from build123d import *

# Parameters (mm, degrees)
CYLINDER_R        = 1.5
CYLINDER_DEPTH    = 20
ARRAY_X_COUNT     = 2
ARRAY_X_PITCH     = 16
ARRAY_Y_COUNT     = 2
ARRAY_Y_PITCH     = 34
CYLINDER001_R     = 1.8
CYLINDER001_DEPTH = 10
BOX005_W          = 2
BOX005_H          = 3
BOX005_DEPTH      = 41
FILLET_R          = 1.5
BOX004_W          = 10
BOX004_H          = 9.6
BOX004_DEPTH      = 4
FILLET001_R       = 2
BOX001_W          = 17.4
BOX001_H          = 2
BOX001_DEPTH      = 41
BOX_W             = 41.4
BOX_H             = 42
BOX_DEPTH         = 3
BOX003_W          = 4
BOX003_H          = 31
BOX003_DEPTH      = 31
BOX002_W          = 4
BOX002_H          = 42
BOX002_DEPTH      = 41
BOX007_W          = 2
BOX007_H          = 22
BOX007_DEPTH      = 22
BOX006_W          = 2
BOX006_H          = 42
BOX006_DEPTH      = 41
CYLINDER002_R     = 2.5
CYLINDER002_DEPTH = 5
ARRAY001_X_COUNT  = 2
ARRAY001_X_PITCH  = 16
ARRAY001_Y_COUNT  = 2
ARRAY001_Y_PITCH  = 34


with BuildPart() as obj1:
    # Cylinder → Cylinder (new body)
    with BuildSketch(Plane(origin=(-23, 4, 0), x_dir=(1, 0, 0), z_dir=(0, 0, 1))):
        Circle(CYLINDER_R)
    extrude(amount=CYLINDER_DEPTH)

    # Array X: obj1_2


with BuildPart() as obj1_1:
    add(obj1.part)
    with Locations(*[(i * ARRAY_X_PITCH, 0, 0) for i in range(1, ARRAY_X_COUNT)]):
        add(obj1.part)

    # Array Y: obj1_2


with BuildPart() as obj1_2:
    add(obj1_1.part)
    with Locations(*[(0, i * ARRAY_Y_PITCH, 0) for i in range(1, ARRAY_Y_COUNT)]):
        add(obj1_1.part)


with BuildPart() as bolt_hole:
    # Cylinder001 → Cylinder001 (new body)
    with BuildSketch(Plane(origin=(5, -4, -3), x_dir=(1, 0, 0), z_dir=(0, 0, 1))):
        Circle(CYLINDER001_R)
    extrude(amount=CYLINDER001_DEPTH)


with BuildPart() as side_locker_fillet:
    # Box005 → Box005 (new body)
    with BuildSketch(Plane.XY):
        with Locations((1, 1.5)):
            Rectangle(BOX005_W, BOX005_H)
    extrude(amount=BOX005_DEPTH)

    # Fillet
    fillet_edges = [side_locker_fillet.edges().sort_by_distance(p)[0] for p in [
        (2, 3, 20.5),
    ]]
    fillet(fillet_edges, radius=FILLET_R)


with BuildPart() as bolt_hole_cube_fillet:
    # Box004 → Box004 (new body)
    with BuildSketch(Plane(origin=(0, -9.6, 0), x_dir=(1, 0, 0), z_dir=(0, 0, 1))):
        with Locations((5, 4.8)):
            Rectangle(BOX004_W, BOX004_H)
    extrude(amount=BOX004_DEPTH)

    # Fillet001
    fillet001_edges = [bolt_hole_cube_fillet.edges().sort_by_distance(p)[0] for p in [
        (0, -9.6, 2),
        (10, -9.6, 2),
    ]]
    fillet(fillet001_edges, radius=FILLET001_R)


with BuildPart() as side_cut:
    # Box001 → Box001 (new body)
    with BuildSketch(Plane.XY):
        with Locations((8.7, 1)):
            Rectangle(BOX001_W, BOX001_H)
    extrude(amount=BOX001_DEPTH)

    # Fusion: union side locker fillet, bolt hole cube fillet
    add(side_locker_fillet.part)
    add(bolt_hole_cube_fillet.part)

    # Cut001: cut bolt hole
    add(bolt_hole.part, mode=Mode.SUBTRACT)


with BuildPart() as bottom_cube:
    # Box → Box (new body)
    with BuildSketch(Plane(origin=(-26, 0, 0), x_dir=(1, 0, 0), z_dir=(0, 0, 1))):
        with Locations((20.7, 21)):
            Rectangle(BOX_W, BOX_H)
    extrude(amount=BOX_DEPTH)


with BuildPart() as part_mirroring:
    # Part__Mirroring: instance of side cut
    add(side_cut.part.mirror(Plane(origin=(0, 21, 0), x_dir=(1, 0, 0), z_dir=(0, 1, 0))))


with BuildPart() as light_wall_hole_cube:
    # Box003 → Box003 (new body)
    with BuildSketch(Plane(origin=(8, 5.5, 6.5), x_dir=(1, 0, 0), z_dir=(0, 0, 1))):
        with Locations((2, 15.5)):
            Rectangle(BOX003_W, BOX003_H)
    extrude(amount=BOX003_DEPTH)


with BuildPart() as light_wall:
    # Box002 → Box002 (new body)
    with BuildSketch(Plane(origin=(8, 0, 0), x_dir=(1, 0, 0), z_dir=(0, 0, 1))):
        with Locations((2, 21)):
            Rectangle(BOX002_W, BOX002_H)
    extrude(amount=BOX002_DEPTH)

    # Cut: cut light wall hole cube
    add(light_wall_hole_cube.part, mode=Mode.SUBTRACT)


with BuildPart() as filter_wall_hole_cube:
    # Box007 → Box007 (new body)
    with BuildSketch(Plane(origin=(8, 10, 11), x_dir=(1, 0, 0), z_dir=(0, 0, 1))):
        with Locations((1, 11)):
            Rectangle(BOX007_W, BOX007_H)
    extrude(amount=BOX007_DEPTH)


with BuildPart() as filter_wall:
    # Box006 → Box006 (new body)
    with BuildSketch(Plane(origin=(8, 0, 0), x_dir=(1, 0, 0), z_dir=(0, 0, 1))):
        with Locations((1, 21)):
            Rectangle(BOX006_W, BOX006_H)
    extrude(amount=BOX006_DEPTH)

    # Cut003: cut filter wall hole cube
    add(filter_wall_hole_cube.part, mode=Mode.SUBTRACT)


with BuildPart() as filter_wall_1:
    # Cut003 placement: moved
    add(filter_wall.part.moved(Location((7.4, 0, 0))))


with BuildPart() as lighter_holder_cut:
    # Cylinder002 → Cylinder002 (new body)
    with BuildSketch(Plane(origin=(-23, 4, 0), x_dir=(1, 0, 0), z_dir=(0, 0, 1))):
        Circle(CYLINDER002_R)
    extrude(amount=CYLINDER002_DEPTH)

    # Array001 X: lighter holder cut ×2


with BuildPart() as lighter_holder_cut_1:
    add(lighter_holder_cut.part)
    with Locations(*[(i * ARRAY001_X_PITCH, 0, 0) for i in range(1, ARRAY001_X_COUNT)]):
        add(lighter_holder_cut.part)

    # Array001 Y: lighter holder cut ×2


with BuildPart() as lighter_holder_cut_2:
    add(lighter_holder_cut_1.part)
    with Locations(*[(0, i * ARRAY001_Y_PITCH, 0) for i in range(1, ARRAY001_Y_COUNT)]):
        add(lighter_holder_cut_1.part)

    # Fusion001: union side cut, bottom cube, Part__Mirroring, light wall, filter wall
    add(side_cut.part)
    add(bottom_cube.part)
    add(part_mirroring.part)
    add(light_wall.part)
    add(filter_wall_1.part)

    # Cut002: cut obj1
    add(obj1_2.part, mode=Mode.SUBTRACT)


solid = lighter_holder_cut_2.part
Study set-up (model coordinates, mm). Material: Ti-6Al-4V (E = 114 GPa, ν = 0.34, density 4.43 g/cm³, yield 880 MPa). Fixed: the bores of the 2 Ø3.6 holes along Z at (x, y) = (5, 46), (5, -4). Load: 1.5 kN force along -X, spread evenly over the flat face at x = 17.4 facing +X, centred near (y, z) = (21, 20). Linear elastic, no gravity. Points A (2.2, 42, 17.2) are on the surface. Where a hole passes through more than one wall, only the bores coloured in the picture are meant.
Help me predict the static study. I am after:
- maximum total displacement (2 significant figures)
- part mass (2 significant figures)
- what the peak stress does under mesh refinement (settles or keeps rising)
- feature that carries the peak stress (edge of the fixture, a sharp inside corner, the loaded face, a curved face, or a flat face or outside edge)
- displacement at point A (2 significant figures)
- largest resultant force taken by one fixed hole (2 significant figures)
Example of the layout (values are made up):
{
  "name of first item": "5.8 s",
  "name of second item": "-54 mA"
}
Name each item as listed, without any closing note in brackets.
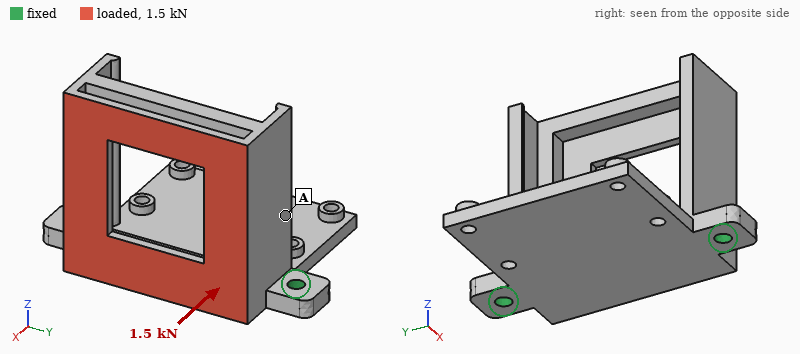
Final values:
{
  "maximum total displacement": "0.45 mm",
  "part mass": "57 g",
  "what the peak stress does under mesh refinement": "keeps rising",
  "feature that carries the peak stress": "edge of the fixture",
  "displacement at point A": "0.13 mm",
  "largest resultant force taken by one fixed hole": "750 N"
}
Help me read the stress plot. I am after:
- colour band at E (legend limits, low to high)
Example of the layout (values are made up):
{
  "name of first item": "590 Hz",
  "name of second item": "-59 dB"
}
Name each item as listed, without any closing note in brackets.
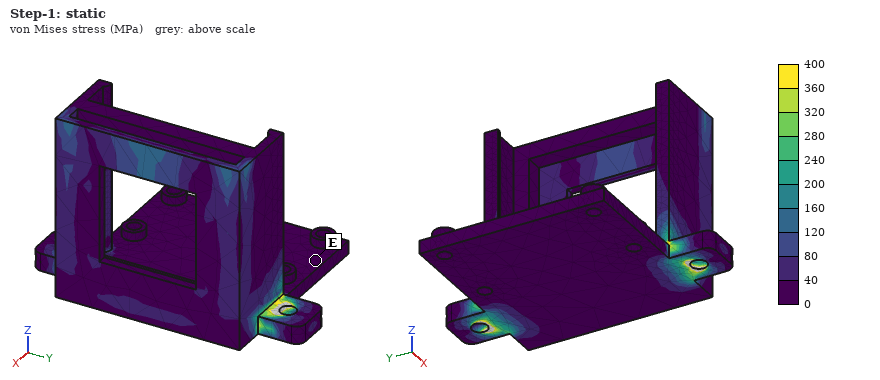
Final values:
{
  "colour band at E": "0 to 40 MPa"
}
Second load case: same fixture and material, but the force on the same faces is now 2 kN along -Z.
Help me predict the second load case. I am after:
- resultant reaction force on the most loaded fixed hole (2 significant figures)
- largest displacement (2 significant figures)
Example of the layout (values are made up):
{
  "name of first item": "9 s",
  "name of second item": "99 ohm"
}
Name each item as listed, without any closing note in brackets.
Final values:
{
  "resultant reaction force on the most loaded fixed hole": "1.0 kN",
  "largest displacement": "0.32 mm"
}
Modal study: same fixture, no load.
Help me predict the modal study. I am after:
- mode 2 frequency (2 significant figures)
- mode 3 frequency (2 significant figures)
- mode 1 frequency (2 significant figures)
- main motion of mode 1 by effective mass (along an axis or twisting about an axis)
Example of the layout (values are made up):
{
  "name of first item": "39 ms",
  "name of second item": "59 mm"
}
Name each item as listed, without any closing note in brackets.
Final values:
{
  "mode 2 frequency": "2800 Hz",
  "mode 3 frequency": "2800 Hz",
  "mode 1 frequency": "1700 Hz",
  "main motion of mode 1 by effective mass": "along X"
}
